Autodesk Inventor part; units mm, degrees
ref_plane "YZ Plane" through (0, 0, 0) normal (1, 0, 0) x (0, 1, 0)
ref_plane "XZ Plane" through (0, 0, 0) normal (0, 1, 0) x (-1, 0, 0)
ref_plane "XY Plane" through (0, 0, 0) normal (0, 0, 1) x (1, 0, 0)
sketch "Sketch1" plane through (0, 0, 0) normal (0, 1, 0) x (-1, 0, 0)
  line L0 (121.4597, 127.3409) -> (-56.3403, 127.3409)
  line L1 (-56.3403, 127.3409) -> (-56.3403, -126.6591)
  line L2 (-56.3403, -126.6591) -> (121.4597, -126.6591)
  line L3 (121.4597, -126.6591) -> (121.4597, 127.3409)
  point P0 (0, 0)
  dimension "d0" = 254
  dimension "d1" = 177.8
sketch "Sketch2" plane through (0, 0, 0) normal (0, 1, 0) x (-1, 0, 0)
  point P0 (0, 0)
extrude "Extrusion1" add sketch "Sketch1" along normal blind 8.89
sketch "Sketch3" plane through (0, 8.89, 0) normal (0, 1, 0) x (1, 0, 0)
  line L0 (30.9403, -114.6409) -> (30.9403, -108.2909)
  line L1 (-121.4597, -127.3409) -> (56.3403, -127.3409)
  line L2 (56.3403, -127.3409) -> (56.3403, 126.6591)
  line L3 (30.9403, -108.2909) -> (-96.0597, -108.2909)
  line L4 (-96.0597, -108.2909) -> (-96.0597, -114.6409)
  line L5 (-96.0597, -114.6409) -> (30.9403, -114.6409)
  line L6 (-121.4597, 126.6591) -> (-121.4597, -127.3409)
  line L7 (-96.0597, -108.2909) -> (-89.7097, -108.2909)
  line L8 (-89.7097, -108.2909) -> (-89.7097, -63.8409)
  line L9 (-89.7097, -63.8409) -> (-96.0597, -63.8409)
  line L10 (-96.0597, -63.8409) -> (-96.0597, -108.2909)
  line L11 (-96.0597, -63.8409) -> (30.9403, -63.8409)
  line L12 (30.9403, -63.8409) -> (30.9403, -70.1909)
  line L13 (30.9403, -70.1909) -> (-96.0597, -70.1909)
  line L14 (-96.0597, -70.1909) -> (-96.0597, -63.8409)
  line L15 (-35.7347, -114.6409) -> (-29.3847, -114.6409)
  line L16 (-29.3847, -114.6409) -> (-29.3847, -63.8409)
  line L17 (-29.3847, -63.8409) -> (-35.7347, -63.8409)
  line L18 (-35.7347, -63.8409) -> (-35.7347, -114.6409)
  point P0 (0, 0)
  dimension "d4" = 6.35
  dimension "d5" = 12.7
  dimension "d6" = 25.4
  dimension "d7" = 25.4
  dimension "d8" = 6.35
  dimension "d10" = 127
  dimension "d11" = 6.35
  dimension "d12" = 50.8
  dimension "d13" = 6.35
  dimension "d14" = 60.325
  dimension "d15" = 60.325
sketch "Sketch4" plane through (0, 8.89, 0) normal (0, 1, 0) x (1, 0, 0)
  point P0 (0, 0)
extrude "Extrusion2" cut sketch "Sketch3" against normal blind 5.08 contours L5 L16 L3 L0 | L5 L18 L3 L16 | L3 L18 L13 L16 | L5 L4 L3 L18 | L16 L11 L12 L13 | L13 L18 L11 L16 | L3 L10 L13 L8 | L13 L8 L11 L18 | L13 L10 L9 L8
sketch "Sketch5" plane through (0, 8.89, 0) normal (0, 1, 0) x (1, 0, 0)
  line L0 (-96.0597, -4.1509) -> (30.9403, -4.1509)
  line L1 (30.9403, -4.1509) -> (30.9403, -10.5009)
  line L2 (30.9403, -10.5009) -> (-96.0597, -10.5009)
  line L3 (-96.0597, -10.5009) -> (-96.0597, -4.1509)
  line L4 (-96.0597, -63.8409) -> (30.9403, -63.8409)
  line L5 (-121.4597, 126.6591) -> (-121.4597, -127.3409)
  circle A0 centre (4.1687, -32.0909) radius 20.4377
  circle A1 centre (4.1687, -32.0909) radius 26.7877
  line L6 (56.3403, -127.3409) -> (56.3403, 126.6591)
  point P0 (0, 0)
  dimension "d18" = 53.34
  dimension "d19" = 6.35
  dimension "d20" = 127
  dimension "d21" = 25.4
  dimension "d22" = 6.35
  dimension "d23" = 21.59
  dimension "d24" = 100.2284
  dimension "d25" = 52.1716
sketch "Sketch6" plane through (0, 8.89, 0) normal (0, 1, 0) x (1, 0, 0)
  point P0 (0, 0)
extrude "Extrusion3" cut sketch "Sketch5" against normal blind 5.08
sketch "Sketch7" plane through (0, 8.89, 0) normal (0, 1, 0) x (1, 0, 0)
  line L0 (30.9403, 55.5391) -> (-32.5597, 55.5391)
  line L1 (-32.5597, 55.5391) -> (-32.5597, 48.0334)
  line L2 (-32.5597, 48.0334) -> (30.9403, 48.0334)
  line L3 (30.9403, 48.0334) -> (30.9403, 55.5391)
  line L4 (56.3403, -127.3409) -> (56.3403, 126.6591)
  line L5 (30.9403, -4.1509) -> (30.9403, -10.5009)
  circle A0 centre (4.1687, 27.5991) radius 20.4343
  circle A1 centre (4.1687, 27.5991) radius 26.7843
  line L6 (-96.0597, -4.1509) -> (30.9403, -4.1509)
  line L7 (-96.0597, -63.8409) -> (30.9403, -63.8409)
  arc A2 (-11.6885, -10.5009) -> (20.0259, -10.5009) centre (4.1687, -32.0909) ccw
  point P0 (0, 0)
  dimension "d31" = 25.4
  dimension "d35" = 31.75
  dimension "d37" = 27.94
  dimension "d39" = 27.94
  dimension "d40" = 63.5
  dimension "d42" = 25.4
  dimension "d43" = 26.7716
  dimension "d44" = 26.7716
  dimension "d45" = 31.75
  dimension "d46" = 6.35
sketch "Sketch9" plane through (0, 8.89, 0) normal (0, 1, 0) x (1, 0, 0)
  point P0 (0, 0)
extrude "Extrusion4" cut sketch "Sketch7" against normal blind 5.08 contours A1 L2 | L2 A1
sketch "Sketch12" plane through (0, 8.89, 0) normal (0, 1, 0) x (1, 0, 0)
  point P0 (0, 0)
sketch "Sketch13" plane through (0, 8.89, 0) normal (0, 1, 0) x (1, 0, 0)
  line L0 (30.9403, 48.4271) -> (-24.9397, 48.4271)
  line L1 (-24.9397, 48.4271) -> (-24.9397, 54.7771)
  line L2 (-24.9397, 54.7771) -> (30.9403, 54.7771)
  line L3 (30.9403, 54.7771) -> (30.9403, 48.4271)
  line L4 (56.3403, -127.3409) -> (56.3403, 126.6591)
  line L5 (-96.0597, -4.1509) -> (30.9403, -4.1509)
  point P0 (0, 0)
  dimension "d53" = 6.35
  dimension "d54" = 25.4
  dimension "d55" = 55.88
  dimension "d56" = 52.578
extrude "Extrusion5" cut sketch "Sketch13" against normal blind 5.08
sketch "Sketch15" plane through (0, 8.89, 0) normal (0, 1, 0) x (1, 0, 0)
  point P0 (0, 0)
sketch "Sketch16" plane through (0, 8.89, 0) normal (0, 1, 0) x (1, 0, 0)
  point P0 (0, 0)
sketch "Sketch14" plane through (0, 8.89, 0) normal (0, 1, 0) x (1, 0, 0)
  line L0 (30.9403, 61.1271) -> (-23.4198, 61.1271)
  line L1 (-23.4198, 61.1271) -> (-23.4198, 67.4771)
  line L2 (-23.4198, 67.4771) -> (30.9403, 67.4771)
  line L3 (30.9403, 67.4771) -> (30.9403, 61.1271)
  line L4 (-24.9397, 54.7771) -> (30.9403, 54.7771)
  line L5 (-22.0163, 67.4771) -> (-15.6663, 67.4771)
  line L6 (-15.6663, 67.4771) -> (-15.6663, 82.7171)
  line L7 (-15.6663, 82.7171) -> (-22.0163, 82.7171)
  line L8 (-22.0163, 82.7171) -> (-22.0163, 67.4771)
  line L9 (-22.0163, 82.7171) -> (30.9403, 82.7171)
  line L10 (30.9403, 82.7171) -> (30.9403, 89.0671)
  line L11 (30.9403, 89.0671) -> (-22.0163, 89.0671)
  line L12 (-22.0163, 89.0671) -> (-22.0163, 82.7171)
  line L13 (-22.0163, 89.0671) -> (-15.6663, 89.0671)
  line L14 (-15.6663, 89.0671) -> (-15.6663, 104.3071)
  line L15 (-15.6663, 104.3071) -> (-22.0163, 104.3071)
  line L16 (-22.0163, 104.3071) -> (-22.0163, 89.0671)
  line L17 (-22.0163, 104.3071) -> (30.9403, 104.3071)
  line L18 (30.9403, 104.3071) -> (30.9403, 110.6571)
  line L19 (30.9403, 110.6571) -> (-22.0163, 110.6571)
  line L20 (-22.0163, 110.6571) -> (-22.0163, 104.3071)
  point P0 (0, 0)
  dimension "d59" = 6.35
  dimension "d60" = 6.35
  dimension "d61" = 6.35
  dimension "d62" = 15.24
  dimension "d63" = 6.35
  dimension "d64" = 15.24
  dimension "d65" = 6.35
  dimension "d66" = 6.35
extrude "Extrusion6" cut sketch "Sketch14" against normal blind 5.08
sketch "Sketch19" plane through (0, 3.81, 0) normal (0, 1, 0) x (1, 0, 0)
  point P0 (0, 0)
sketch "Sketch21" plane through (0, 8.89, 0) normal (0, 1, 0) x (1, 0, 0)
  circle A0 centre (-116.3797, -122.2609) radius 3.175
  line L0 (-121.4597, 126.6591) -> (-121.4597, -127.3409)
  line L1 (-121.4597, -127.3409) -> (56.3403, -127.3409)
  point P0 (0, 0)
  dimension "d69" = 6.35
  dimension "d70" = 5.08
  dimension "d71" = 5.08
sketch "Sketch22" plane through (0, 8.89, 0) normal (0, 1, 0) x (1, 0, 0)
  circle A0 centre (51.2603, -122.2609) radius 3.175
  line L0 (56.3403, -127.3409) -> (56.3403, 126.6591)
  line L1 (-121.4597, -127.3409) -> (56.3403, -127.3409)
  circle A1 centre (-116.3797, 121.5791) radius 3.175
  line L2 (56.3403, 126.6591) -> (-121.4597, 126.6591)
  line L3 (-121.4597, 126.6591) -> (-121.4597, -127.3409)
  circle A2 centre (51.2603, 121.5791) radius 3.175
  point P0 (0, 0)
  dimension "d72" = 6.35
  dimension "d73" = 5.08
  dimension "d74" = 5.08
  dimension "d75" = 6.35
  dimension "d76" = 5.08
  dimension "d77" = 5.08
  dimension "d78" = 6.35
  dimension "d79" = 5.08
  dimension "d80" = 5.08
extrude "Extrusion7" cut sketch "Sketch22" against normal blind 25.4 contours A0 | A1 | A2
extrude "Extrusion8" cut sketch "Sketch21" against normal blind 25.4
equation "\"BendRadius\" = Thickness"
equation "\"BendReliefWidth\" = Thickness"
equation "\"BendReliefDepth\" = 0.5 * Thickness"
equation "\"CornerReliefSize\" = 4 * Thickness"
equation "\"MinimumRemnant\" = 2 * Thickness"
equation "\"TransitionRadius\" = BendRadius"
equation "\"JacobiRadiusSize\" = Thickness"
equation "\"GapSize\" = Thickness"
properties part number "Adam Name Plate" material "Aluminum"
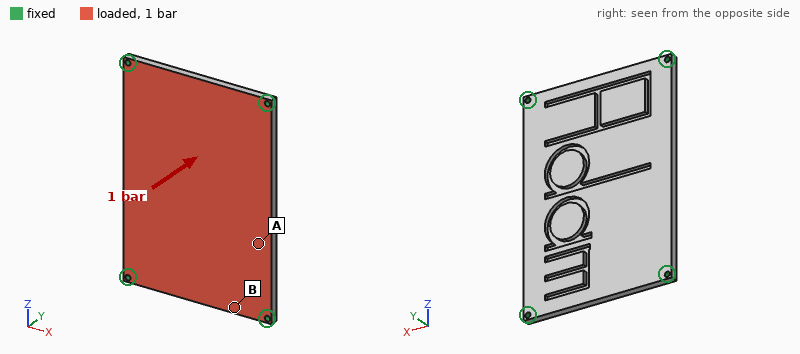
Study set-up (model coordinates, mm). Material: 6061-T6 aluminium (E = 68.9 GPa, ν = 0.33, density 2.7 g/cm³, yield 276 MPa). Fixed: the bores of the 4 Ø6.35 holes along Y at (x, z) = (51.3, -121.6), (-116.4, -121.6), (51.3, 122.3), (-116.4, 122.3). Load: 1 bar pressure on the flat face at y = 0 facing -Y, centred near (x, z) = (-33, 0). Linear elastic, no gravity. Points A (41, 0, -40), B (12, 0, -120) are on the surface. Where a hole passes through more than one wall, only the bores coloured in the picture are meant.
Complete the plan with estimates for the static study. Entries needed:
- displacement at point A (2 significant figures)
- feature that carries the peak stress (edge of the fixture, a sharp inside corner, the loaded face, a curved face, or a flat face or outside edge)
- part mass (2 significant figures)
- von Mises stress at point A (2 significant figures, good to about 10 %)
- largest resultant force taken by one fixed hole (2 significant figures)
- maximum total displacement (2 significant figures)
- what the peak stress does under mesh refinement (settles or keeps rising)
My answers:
0.48 mm
edge of the fixture
1000 g
25 MPa
1.9 kN
0.69 mm
keeps rising
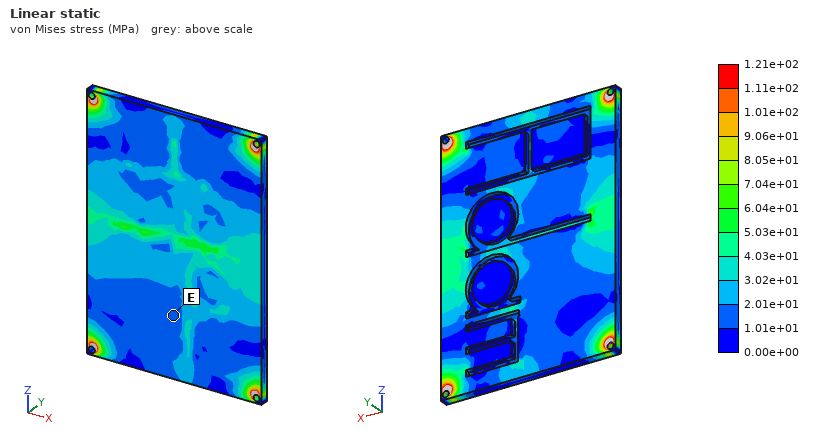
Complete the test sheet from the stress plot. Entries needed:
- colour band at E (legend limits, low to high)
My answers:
1.01e+01 to 2.01e+01 MPa
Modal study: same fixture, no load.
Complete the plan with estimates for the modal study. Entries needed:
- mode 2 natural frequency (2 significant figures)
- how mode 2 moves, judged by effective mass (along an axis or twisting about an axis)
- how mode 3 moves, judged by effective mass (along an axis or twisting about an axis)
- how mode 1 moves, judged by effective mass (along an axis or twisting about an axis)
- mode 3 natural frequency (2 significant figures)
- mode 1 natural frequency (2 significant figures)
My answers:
900 Hz
twisting about Z
twisting about X
along Y
1200 Hz
490 Hz
